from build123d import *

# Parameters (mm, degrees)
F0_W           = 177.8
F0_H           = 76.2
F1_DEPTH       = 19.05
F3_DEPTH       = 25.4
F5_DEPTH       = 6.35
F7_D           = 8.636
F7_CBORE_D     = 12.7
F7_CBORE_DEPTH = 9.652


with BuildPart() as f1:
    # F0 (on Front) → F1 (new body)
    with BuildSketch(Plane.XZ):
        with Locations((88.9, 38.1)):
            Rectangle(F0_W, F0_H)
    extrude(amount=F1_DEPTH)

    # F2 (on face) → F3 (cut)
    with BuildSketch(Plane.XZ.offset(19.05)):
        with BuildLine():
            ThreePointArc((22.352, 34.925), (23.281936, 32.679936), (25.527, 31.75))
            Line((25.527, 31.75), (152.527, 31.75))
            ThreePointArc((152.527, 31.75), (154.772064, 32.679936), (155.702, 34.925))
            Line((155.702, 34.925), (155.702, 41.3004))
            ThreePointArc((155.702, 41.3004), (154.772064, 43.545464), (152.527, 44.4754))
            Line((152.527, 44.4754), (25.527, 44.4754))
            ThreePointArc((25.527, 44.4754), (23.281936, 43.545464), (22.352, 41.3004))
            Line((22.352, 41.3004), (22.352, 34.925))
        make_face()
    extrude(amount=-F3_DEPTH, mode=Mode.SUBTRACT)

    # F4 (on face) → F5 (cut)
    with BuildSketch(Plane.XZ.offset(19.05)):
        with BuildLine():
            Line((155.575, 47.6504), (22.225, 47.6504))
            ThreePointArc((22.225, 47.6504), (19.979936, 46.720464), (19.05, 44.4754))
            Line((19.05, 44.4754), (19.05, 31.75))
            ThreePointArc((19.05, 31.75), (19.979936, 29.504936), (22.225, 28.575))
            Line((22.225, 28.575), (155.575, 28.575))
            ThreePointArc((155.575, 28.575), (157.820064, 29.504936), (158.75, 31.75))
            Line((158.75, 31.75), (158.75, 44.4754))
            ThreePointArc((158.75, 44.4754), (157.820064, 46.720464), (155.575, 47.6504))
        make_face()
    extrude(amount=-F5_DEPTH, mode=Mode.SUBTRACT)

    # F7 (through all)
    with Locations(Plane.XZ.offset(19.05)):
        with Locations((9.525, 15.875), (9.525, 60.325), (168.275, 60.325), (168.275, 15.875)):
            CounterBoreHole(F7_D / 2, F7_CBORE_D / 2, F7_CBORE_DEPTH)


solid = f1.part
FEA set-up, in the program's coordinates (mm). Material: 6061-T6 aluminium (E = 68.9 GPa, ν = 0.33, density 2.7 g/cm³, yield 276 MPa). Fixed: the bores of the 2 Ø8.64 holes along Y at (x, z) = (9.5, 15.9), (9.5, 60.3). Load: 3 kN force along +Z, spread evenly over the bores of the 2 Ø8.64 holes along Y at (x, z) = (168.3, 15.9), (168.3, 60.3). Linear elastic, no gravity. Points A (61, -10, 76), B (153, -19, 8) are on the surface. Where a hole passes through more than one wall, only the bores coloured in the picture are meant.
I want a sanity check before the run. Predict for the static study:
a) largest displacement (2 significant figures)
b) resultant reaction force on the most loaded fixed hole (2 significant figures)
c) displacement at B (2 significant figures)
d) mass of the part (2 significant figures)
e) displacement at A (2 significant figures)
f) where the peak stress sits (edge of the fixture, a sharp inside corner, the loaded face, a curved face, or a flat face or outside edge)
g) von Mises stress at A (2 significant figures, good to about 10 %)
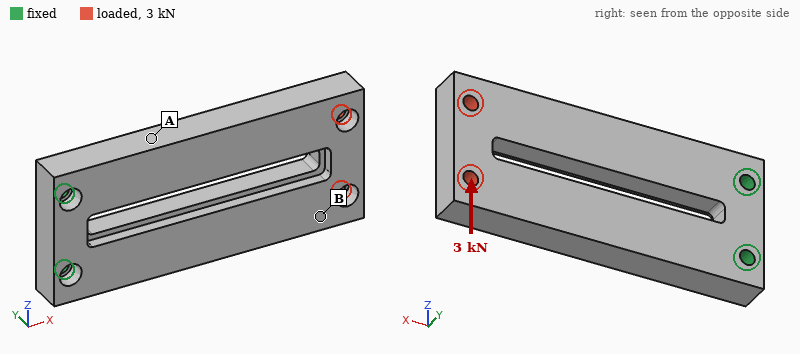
0.34 mm
9.0 kN
0.28 mm
570 g
0.091 mm
edge of the fixture
27 MPa
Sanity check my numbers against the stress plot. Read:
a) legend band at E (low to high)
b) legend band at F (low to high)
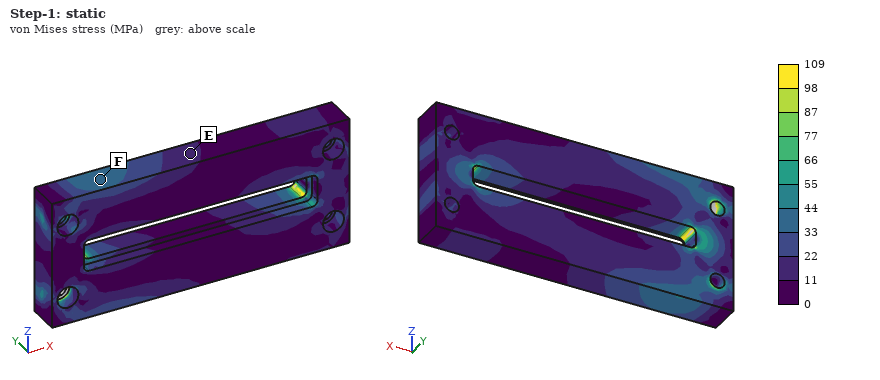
11 to 22 MPa
33 to 44 MPa
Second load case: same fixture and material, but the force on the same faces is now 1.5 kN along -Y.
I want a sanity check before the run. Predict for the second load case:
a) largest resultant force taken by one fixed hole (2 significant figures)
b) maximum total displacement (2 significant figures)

820 N
1.3 mm
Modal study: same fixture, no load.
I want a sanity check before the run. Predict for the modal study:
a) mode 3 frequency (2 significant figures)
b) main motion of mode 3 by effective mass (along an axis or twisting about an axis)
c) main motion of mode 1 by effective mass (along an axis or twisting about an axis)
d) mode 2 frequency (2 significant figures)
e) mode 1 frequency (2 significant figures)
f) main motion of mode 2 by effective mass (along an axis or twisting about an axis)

1700 Hz
twisting about X
along Y
1100 Hz
430 Hz
along Z
